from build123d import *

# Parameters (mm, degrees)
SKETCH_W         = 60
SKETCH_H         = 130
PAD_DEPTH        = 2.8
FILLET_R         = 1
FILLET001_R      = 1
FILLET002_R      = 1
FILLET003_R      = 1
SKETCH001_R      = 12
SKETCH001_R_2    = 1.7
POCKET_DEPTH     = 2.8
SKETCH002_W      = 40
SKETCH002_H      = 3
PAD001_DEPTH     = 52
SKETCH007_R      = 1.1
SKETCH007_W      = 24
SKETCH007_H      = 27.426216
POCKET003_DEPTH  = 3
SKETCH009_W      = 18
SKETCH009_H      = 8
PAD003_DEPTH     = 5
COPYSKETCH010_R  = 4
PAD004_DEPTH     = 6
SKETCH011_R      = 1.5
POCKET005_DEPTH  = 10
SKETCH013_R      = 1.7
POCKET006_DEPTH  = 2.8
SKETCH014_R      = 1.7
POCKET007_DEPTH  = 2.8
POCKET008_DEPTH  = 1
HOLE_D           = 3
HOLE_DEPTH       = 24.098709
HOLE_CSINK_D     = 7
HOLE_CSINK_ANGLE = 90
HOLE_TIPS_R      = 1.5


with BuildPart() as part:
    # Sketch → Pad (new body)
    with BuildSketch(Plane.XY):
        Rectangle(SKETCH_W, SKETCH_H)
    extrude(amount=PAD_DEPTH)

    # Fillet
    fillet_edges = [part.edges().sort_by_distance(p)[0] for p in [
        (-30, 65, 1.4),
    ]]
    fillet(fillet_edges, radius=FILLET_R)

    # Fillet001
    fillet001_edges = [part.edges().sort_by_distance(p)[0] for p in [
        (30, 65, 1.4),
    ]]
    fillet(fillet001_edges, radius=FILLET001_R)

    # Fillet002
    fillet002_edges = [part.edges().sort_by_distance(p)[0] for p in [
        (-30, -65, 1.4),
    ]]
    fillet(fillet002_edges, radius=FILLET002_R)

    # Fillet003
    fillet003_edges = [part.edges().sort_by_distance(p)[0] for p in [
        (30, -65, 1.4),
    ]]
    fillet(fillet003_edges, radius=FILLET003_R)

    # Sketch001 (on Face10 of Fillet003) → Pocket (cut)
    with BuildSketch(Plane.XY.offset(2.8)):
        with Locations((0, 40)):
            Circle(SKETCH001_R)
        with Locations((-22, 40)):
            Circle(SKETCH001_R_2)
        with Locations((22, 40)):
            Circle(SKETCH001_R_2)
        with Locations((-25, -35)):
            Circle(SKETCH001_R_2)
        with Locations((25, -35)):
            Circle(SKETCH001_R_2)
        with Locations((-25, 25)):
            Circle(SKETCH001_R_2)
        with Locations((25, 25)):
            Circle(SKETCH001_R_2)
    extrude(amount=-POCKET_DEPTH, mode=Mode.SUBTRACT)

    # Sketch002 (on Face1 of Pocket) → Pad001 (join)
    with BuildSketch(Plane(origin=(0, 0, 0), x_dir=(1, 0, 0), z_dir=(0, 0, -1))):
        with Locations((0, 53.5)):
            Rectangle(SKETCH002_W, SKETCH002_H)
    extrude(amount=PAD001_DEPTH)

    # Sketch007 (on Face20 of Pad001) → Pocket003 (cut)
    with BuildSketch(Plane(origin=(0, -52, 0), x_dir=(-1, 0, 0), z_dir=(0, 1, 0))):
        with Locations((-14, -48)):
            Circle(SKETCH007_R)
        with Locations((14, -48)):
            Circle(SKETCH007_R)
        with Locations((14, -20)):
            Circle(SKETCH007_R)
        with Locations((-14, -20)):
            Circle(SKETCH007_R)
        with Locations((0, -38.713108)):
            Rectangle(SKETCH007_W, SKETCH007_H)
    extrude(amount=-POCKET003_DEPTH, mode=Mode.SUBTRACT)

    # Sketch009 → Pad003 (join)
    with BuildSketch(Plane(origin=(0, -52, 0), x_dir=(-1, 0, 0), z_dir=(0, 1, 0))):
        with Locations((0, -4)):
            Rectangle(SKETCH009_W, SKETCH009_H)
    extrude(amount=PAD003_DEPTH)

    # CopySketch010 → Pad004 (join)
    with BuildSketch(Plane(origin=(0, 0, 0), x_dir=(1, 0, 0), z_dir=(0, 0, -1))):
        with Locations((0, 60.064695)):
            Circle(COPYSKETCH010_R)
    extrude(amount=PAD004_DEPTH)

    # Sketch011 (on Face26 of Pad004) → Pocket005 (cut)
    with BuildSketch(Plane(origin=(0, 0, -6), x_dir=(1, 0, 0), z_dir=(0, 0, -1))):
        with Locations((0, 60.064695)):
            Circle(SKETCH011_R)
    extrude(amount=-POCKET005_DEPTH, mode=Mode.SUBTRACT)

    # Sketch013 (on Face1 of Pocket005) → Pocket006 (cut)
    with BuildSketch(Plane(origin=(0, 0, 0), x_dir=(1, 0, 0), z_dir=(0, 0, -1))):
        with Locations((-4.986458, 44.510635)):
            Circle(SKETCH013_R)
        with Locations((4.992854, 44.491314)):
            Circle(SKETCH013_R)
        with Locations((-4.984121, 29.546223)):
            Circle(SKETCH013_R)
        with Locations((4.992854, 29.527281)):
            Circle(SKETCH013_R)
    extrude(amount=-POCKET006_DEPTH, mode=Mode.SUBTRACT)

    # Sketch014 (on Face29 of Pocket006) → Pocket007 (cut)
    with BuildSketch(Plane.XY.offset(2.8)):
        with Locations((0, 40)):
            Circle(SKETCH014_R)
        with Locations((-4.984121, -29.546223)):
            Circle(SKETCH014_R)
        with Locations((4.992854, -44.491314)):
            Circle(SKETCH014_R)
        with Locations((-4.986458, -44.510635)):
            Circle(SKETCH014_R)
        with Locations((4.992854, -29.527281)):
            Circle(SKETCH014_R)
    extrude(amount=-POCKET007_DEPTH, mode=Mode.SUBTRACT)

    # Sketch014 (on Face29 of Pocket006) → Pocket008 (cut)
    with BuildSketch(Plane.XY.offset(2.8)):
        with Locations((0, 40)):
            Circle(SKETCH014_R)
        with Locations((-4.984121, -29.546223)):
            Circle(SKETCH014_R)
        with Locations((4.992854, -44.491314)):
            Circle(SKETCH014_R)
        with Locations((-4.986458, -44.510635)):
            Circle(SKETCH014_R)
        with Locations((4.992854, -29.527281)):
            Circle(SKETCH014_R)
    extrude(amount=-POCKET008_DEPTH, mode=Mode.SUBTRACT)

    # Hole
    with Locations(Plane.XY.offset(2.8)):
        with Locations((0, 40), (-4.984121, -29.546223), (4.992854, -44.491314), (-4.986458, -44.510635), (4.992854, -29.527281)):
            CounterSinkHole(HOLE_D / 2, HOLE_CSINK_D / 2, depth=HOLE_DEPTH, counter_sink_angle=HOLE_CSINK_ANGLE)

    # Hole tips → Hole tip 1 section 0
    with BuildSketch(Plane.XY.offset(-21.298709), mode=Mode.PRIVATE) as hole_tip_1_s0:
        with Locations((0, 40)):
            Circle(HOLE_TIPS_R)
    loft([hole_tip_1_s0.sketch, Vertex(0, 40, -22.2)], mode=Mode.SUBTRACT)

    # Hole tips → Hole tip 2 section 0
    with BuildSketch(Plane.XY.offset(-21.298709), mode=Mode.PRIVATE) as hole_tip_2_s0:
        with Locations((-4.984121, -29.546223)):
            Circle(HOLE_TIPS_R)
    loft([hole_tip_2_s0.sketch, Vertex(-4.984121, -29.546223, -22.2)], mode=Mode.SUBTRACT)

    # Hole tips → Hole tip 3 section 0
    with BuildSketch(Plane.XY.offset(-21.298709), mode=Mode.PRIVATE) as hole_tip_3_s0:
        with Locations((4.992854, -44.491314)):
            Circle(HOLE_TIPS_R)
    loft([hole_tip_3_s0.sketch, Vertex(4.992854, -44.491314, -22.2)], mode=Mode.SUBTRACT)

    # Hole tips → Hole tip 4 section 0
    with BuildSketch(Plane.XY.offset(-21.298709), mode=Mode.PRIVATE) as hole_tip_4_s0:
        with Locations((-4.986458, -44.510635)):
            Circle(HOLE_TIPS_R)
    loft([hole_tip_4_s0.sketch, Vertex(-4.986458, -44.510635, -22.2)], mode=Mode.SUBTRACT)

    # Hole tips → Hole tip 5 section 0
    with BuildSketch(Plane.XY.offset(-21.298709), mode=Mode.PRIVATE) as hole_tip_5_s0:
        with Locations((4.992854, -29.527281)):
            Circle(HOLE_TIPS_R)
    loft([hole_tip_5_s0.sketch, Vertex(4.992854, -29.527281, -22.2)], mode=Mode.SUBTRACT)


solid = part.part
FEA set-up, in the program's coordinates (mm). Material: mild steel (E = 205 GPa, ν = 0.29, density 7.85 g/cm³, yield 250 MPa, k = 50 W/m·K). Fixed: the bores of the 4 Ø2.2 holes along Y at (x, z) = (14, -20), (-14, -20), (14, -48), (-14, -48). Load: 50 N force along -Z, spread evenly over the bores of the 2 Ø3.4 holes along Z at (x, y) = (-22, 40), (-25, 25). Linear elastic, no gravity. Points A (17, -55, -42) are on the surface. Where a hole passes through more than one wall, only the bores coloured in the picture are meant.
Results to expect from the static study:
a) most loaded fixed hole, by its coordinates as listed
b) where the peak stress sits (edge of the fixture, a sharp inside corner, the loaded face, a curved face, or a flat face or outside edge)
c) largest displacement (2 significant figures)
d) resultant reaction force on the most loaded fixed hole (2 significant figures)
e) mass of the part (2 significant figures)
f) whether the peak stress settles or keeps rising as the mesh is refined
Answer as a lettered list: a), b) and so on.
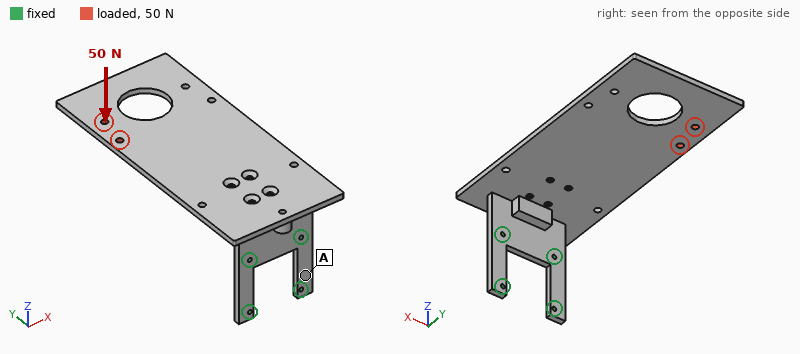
a) (-14, -20)
b) edge of the fixture
c) 1.3 mm
d) 70 N
e) 200 g
f) keeps rising
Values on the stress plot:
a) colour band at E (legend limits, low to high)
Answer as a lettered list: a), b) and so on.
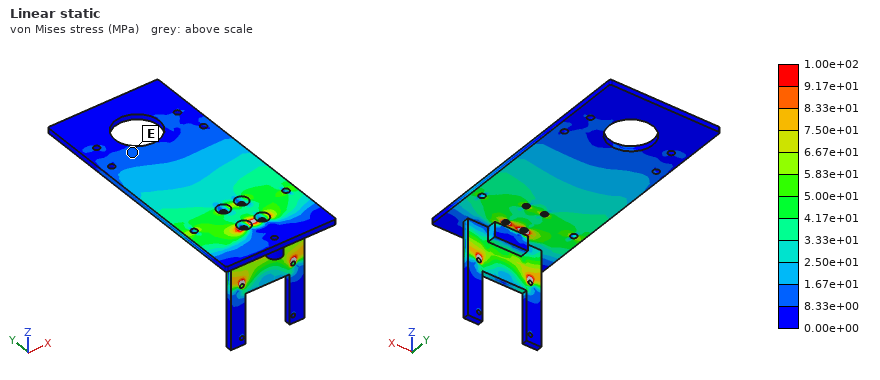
a) 8.33e+00 to 1.67e+01 MPa
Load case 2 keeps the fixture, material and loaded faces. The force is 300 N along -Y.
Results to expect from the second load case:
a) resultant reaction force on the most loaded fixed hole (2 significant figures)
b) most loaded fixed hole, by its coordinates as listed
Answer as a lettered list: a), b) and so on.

a) 420 N
b) (-14, -20)
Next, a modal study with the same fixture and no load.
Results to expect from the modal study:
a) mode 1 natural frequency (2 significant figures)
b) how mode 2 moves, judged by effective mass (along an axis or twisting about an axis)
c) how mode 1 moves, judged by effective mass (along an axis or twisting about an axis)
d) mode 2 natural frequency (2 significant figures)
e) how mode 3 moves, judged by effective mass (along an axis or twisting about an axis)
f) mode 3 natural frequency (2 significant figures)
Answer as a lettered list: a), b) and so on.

a) 140 Hz
b) along X
c) along Z
d) 430 Hz
e) twisting about Y
f) 670 Hz
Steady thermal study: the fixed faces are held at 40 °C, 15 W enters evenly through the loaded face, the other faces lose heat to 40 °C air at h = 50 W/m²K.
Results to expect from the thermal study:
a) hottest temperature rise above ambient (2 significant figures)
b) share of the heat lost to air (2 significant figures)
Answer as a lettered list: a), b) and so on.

a) 74 K
b) 95 %
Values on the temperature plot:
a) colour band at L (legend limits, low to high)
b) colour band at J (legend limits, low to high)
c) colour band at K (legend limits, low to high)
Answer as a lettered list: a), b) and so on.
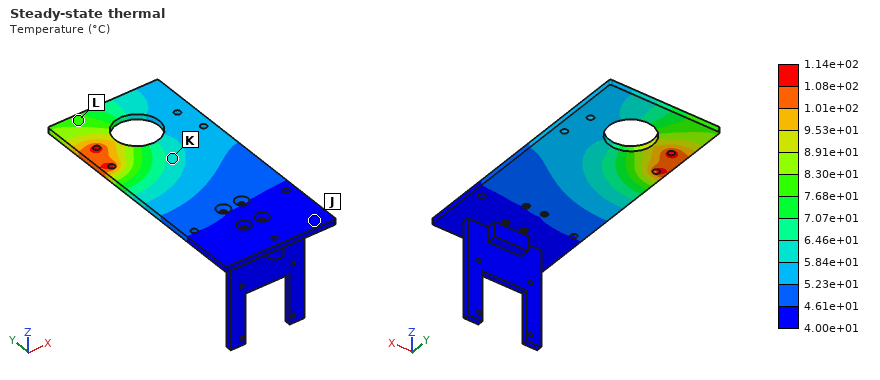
a) 7.68e+01 to 8.30e+01 °C
b) 4.00e+01 to 4.61e+01 °C
c) 5.84e+01 to 6.46e+01 °C
